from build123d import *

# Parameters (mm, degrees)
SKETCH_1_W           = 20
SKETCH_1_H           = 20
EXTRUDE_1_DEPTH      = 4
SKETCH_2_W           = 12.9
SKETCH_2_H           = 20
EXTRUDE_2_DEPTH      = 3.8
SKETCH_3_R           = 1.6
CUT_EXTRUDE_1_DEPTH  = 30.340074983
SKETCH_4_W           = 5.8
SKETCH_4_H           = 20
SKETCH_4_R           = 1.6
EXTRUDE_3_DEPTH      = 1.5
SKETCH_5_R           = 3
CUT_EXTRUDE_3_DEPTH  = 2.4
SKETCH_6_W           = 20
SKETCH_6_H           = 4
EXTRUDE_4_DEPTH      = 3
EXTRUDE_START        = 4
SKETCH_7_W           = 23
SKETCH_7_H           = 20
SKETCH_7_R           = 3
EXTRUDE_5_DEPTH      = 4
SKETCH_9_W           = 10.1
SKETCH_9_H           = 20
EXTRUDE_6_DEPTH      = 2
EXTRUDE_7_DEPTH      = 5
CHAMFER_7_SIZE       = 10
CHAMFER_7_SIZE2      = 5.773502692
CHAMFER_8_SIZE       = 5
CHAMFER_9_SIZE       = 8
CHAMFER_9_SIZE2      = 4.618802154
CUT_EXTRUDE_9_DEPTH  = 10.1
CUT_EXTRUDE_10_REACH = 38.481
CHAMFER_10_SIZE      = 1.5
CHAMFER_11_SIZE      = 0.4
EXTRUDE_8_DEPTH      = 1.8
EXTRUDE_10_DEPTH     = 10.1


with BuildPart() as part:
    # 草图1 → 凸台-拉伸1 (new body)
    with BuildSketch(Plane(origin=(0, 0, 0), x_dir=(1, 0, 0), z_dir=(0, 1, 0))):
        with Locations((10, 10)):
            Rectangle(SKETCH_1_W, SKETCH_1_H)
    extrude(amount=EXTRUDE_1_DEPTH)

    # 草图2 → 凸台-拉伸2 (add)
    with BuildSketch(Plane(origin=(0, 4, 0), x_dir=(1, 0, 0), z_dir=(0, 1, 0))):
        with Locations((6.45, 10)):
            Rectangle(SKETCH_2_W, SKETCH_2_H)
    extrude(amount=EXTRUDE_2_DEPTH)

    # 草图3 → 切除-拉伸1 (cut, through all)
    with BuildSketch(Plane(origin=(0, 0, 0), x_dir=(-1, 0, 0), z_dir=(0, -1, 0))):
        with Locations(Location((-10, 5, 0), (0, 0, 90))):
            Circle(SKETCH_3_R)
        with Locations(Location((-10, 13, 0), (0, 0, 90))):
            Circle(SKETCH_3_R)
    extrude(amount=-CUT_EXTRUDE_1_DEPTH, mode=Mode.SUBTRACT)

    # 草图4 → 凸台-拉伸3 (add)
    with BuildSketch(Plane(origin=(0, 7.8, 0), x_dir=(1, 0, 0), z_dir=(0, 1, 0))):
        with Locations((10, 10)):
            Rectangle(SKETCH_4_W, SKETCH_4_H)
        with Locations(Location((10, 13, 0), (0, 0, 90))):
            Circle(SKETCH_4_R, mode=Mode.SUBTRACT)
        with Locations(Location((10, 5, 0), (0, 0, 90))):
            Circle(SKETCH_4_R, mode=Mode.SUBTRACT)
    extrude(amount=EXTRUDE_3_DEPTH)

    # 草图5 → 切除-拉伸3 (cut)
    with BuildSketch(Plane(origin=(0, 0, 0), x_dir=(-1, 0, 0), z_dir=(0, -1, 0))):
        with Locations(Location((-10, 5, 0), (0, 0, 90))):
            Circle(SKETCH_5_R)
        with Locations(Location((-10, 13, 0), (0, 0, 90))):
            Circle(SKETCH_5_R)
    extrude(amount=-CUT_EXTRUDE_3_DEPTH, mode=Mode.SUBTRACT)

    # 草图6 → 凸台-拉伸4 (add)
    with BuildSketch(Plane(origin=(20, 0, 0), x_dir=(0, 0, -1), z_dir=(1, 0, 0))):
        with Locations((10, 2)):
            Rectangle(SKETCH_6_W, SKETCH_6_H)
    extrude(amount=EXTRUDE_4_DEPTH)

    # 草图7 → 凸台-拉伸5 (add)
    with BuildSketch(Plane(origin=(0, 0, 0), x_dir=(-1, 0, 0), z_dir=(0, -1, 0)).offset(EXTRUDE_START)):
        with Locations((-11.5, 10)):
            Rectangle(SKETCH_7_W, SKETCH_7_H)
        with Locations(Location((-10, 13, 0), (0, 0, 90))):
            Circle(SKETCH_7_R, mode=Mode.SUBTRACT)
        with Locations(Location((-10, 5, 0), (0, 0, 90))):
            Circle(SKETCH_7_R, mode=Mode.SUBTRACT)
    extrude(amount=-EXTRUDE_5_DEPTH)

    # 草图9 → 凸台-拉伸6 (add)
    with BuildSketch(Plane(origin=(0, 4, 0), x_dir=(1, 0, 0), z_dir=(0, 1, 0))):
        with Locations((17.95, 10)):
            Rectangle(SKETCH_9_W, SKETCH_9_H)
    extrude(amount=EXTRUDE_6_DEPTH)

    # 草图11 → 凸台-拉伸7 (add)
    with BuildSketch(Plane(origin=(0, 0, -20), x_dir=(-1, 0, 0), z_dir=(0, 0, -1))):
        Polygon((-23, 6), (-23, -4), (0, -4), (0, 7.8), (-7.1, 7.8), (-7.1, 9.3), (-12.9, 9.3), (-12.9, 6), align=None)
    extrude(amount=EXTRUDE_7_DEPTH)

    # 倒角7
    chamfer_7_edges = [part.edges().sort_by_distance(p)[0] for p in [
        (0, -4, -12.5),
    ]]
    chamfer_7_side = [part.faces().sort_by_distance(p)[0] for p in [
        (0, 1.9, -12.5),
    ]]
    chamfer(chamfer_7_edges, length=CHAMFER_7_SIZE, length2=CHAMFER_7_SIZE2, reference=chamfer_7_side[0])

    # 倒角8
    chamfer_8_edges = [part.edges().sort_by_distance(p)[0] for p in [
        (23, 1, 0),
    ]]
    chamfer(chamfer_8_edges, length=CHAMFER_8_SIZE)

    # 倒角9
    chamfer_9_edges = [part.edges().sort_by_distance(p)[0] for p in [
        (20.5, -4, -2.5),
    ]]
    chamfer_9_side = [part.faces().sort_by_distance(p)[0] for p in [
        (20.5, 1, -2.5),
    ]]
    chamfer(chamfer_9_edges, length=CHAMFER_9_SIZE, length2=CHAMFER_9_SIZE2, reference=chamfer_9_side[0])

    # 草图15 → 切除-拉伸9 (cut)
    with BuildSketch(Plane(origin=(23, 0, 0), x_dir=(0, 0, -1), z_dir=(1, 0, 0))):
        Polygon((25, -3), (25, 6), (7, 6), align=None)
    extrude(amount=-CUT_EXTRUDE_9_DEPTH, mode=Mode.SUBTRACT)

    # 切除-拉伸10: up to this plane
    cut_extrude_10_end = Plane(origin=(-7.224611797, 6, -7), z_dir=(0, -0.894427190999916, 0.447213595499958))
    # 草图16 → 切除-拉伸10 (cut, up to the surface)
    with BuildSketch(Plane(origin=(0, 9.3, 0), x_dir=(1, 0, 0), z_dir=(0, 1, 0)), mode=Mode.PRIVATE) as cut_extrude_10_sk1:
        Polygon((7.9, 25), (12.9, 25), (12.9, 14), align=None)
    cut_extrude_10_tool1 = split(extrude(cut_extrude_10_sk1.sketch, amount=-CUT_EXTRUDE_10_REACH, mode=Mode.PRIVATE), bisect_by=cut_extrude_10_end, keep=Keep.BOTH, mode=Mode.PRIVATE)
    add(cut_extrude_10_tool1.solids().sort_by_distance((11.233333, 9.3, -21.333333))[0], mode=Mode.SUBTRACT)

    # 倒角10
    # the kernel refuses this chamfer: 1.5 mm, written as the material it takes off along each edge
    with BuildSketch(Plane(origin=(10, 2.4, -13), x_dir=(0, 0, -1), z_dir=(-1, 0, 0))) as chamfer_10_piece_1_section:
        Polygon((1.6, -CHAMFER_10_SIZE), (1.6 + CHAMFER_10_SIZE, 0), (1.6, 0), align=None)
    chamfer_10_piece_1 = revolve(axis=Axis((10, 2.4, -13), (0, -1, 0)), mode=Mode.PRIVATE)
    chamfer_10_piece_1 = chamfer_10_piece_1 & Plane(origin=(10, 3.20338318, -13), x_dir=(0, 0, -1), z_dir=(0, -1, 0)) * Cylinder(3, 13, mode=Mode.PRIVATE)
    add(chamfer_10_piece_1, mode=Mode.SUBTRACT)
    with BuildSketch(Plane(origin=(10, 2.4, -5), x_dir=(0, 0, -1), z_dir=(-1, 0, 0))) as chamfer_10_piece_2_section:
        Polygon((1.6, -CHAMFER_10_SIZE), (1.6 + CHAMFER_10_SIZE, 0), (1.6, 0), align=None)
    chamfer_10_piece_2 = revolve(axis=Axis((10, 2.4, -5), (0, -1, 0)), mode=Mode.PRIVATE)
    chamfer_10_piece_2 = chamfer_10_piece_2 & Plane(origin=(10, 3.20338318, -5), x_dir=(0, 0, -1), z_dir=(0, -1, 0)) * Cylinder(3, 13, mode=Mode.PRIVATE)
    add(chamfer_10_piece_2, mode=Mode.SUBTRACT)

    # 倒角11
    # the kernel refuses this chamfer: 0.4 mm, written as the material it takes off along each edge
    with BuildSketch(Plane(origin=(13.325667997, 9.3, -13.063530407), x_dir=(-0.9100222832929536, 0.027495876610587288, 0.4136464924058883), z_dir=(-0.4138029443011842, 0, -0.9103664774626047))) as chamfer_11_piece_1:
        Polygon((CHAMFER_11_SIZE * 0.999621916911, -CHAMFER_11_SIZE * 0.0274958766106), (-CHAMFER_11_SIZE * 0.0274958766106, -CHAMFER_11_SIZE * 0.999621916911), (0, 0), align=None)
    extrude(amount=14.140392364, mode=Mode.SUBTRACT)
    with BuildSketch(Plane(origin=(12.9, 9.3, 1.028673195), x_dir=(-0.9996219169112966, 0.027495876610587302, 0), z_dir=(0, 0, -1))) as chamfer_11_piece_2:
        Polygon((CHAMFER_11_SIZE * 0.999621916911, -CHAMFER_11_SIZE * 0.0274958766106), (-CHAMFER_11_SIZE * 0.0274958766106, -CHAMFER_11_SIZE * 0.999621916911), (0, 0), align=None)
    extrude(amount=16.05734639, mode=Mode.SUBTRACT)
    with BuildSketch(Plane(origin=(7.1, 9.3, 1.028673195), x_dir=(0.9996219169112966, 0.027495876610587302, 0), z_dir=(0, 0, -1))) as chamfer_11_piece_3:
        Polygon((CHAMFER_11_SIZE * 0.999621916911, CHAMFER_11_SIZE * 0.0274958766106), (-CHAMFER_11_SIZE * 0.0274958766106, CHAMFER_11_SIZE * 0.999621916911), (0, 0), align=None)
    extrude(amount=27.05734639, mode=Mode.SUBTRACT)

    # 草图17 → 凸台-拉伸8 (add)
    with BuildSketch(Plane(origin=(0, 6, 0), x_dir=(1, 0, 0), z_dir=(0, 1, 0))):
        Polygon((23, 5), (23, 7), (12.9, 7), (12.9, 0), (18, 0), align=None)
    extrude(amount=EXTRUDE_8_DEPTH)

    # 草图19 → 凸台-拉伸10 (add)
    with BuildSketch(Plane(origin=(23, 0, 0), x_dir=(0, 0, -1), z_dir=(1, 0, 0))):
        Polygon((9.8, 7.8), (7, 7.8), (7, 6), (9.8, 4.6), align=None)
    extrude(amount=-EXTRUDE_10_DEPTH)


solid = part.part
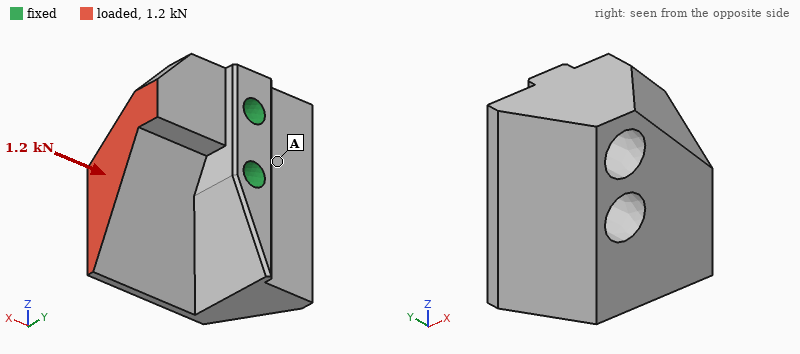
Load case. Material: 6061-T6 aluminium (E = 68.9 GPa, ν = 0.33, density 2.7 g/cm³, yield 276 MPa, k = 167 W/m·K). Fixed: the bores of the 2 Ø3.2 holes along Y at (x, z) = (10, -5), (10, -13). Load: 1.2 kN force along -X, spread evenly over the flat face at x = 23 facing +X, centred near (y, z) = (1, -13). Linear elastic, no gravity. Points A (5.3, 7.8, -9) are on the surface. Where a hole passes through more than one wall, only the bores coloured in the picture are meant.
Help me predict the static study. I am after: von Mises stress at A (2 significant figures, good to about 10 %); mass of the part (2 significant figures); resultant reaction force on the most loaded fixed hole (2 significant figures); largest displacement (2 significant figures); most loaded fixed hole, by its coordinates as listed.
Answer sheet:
18 MPa
11 g
1.0 kN
24 µm
(10, -13)
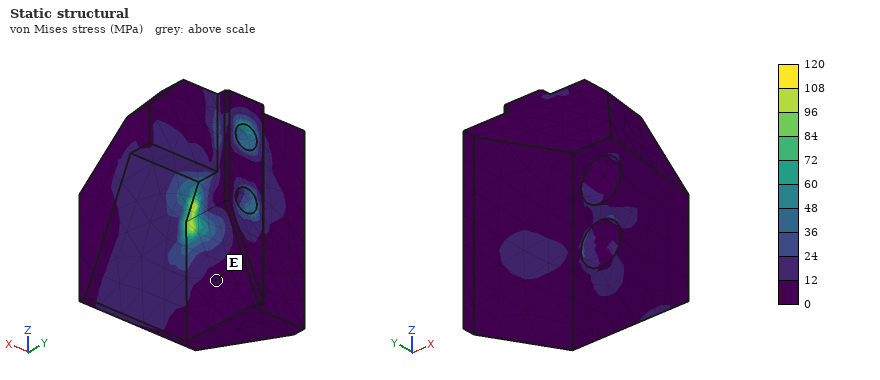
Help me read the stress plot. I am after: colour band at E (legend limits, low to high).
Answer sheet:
0 to 12 MPa
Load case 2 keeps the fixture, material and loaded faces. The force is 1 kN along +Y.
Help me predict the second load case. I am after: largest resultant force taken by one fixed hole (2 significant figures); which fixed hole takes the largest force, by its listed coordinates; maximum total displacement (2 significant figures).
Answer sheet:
800 N
(10, -13)
77 µm
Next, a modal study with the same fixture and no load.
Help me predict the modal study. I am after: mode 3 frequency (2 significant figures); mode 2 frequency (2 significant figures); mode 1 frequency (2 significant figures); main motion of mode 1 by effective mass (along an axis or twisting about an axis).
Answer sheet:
26 kHz
20 kHz
16 kHz
along X
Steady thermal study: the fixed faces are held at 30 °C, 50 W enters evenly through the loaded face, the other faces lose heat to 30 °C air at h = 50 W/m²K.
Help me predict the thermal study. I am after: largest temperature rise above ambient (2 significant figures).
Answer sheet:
44 K
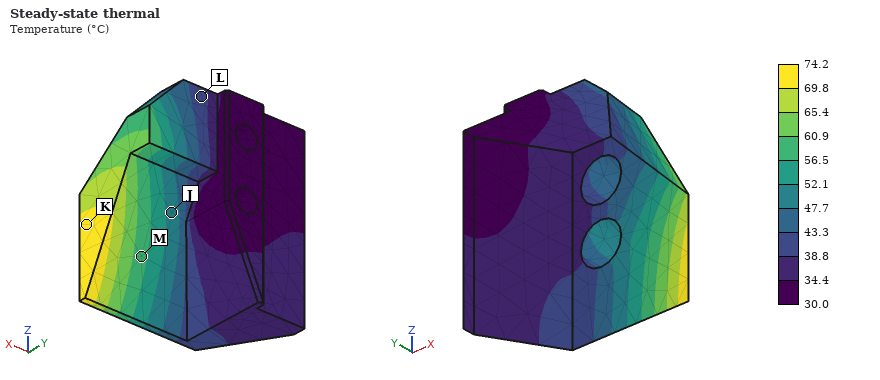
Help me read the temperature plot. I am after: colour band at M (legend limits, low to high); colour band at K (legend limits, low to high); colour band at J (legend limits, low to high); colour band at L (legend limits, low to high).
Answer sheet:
56.5 to 60.9 °C
69.8 to 74.2 °C
47.7 to 52.1 °C
38.8 to 43.3 °C
